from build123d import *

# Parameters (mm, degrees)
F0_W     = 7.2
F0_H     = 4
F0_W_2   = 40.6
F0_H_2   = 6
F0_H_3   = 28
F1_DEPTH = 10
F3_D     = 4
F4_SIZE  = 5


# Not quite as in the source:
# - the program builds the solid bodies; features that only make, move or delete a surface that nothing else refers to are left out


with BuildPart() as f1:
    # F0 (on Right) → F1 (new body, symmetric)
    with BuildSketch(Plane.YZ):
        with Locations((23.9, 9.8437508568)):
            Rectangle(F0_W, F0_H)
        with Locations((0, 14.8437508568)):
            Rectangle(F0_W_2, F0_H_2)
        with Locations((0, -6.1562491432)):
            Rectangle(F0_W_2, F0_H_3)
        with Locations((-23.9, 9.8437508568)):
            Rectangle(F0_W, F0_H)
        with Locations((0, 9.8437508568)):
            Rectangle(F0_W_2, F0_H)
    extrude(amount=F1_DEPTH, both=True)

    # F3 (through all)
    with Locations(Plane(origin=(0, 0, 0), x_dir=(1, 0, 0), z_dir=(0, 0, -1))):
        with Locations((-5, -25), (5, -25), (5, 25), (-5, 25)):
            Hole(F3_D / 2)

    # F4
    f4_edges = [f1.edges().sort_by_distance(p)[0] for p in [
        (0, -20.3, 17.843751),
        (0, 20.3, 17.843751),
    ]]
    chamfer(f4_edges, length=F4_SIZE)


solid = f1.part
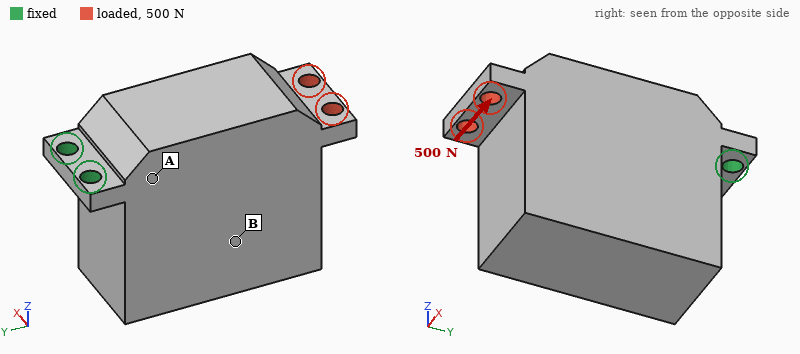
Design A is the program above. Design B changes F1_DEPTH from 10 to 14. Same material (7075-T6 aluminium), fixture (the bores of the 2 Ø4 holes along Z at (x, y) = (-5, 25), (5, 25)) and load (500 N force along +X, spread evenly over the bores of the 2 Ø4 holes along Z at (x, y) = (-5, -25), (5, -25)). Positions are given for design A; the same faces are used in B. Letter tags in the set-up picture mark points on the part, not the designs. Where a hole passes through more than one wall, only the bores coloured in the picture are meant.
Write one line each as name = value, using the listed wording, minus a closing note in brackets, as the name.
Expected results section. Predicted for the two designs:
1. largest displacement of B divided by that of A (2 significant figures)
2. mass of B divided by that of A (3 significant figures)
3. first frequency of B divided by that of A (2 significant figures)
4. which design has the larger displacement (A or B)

largest displacement of B divided by that of A = 0.76
mass of B divided by that of A = 1.40
first frequency of B divided by that of A = 0.92
which design has the larger displacement = A
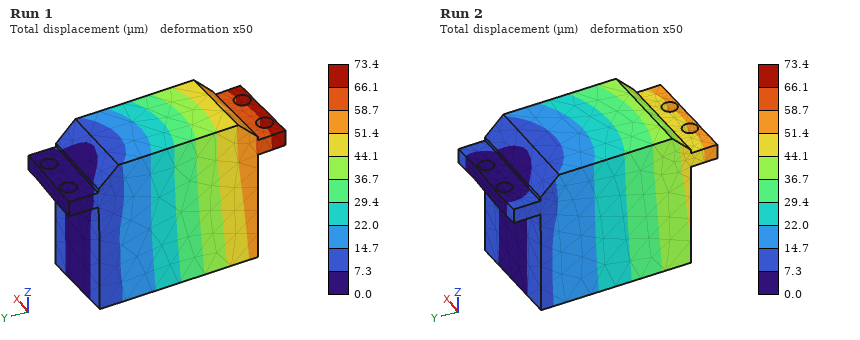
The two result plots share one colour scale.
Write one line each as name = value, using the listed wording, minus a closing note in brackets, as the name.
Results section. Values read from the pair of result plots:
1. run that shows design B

run that shows design B = Run 2
